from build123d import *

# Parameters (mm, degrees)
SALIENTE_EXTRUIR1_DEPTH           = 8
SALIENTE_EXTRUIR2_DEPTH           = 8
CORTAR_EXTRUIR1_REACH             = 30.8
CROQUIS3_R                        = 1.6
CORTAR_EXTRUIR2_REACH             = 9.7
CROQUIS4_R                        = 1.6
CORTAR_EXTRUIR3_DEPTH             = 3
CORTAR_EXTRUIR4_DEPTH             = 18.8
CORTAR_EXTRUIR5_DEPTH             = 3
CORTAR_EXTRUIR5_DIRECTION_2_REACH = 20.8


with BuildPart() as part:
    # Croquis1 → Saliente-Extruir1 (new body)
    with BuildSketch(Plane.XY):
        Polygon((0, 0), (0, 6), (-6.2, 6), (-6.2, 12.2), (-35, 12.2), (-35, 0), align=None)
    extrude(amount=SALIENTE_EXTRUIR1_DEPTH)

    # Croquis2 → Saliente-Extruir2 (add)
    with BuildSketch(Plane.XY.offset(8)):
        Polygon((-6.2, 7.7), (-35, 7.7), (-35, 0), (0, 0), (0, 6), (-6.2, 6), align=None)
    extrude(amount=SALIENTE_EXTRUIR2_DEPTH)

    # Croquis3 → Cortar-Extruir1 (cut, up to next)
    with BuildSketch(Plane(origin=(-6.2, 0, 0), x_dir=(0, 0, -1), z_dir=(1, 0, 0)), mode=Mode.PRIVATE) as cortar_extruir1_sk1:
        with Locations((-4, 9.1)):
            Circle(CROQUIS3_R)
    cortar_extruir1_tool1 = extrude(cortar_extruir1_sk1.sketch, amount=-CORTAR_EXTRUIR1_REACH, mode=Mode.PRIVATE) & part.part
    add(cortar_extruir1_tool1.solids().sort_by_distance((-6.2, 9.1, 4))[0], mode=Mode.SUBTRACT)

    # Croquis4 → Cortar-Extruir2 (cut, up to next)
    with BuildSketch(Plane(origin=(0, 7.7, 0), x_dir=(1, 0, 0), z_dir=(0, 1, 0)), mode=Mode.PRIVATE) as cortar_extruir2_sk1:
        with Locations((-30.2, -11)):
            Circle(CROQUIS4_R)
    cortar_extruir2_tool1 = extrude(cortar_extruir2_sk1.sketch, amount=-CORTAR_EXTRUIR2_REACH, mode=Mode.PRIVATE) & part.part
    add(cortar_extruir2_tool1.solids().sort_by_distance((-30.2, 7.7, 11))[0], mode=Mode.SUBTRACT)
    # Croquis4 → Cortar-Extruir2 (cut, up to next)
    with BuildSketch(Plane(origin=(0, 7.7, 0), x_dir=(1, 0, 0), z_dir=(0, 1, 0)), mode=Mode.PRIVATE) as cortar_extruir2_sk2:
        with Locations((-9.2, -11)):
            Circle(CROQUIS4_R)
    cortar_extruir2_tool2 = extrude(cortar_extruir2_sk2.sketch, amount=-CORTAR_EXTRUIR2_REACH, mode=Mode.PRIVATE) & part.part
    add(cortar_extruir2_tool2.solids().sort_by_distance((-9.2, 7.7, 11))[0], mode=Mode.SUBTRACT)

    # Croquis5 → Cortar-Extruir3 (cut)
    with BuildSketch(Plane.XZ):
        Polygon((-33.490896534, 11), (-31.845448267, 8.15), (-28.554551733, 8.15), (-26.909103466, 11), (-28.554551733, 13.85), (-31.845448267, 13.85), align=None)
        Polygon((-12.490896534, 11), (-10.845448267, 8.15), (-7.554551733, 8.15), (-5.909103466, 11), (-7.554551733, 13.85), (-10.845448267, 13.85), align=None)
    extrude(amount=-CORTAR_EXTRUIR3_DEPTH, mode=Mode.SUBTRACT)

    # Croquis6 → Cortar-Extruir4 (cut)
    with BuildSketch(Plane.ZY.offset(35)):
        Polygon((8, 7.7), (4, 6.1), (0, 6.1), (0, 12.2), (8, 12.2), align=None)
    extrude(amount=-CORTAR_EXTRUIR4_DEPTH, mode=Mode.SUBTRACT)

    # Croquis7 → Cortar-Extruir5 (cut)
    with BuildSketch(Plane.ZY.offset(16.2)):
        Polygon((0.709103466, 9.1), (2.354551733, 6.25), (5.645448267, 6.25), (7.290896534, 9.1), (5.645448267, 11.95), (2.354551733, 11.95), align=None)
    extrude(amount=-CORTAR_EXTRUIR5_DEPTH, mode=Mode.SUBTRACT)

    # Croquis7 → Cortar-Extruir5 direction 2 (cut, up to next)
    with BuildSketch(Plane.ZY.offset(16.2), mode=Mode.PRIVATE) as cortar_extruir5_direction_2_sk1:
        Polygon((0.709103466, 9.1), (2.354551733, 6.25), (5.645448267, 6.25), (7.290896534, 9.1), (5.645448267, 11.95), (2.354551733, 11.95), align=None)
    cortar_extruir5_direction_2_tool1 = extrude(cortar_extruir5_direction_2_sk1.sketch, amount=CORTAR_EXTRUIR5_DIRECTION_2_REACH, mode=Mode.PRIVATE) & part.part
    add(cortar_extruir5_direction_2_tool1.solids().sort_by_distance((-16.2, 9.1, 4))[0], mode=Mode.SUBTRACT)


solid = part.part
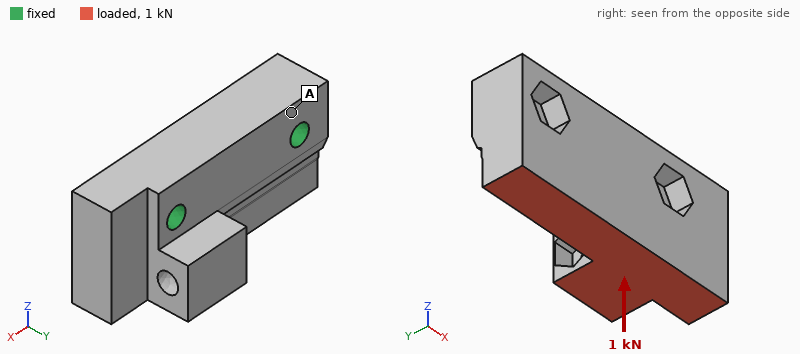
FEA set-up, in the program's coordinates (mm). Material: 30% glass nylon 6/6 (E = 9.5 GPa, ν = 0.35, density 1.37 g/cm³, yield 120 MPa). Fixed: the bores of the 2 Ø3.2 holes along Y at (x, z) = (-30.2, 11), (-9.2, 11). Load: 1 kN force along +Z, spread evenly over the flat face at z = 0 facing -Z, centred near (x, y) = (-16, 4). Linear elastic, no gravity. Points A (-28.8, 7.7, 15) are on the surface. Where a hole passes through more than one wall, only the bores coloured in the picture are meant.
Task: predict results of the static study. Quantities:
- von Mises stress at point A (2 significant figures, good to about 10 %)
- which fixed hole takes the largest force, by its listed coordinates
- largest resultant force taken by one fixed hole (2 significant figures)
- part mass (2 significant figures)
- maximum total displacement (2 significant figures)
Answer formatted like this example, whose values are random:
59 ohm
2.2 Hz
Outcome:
2.5 MPa
(-9.2, 11)
670 N
5.4 g
32 µm
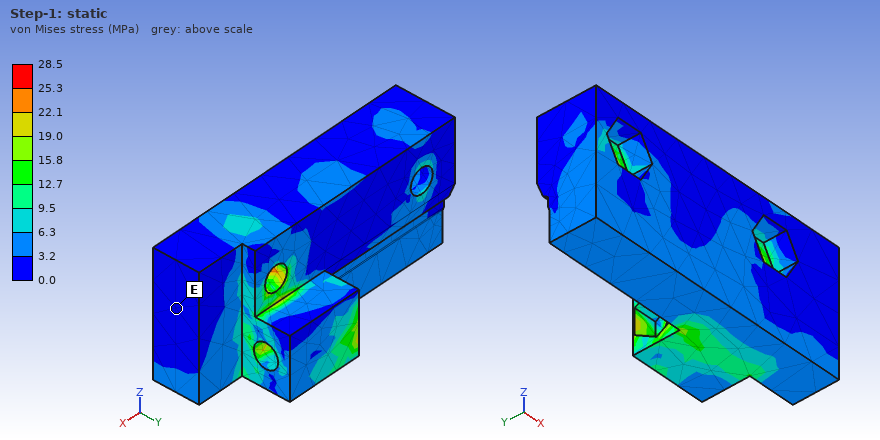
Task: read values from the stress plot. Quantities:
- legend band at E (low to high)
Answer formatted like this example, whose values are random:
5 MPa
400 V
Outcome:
0.0 to 3.2 MPa
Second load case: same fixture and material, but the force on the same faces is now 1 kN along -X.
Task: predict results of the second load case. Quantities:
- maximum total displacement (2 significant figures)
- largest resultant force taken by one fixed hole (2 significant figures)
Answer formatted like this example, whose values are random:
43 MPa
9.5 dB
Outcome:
72 µm
710 N
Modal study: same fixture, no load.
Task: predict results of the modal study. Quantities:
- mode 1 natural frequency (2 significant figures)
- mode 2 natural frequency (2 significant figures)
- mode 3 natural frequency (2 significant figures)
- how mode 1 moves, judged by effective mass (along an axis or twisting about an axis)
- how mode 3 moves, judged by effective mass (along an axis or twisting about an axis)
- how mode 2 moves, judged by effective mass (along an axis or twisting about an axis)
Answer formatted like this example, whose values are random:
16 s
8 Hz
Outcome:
10 kHz
14 kHz
19 kHz
along Y
along X
twisting about Z
